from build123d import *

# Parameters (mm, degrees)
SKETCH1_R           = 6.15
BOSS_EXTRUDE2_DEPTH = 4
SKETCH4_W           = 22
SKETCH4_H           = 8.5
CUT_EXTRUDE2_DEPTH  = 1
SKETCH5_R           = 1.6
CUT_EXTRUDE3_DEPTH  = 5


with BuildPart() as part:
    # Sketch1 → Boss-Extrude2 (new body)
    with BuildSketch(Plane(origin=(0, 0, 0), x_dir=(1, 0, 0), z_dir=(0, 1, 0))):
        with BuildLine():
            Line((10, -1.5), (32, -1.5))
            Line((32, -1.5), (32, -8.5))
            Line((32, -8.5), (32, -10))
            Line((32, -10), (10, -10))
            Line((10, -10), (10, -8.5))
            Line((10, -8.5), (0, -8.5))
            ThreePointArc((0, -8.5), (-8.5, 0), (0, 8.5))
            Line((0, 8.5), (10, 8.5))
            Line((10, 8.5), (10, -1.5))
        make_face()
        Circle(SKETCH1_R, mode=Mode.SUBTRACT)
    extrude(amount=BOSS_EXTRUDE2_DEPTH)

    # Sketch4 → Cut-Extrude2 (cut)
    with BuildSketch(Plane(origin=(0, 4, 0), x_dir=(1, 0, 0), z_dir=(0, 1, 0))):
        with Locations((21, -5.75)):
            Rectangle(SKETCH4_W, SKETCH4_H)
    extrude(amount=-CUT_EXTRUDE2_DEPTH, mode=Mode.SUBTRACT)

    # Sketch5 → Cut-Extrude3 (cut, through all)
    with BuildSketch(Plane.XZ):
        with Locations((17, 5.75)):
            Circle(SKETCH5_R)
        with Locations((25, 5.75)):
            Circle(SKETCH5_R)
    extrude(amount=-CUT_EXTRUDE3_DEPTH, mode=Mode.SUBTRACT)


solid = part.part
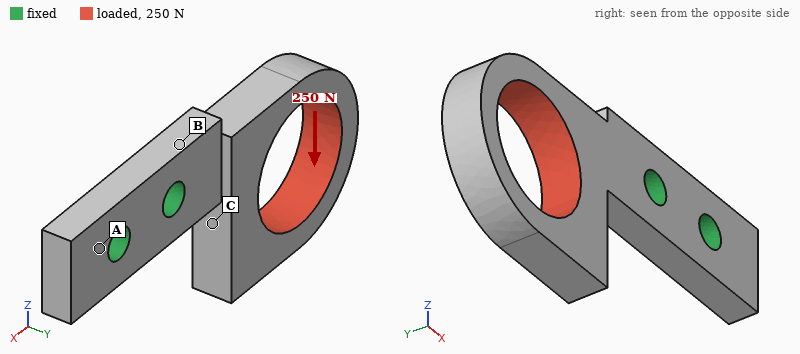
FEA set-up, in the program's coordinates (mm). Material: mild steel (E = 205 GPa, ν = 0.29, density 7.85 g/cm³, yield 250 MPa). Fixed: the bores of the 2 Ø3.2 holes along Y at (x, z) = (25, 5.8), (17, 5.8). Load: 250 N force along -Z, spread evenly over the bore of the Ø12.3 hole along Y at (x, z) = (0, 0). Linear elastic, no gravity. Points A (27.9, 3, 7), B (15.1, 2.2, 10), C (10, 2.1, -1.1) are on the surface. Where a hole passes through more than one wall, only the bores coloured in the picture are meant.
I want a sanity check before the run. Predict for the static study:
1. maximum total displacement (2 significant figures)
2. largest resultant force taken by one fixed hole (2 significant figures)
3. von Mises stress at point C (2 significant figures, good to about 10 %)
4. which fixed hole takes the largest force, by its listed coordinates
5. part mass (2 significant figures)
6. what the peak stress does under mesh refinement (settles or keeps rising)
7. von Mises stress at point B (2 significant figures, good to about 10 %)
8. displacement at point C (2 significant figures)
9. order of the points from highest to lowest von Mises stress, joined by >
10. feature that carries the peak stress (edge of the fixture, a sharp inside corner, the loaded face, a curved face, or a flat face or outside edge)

47 µm
440 N
50 MPa
(17, 5.8)
9.2 g
keeps rising
92 MPa
11 µm
B > C > A
a sharp inside corner
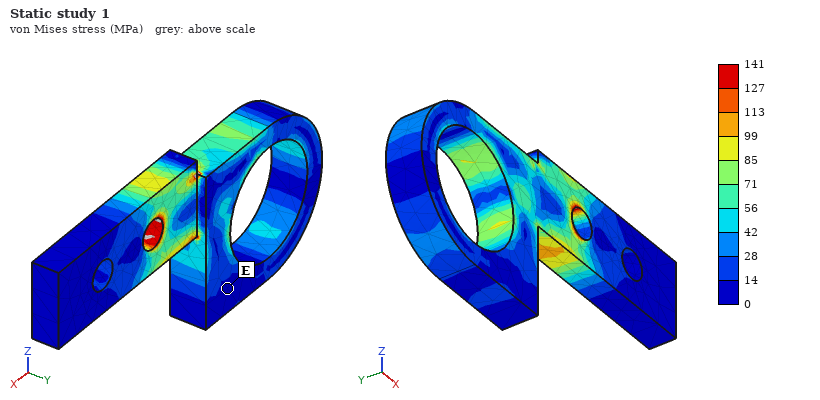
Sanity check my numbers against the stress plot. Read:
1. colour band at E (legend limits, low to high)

0 to 14 MPa
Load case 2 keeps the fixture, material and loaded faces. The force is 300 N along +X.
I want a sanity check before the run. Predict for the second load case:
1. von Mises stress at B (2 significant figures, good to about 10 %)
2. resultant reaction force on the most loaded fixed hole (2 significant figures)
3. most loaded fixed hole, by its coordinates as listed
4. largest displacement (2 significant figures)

32 MPa
280 N
(17, 5.8)
28 µm
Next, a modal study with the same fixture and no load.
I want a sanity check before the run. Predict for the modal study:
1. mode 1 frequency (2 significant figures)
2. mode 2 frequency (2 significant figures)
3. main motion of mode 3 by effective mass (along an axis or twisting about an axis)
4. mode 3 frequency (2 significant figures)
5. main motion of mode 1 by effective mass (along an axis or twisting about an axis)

3600 Hz
6200 Hz
twisting about X
8200 Hz
along Y
